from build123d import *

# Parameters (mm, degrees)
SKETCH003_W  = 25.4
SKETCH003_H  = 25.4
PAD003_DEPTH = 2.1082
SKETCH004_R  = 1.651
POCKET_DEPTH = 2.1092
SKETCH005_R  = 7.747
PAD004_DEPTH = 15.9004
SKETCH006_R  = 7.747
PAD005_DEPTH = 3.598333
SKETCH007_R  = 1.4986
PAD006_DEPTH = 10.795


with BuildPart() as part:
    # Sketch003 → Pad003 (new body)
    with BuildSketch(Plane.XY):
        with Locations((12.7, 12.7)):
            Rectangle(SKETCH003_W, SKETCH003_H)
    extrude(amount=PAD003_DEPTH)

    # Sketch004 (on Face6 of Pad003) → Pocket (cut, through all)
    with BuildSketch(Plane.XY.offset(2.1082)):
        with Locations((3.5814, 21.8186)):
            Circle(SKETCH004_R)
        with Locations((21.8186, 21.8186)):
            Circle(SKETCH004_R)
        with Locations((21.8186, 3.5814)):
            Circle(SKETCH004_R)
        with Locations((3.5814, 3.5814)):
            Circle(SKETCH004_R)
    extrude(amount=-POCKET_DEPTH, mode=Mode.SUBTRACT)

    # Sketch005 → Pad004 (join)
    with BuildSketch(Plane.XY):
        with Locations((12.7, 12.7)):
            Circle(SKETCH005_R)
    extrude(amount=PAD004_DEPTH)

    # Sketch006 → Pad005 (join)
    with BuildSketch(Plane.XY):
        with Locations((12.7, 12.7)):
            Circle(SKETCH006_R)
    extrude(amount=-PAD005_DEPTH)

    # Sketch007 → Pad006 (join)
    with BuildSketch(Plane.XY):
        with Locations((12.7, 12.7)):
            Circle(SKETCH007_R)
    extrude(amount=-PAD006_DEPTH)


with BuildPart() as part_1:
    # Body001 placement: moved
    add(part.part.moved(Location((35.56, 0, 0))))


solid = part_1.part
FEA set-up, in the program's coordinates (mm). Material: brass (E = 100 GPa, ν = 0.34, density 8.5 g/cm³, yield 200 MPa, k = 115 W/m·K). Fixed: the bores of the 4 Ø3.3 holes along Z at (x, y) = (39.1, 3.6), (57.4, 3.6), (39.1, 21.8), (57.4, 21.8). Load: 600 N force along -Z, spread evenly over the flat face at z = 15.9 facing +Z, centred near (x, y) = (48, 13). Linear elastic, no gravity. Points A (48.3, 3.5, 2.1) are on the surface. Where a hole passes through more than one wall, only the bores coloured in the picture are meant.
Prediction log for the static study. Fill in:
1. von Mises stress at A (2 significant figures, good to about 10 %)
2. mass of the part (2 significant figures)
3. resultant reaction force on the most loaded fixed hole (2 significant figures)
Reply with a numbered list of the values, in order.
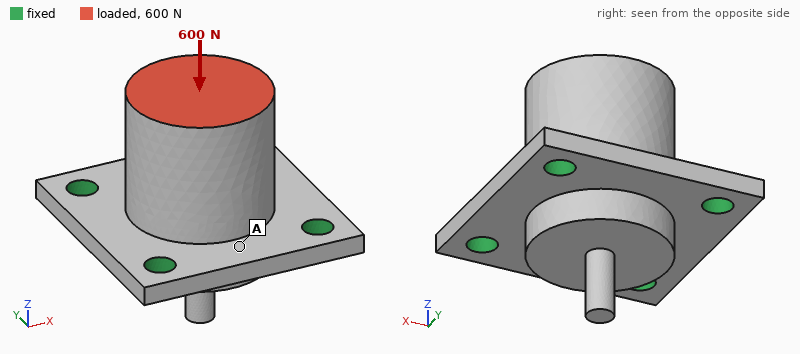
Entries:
1. 12 MPa
2. 39 g
3. 150 N
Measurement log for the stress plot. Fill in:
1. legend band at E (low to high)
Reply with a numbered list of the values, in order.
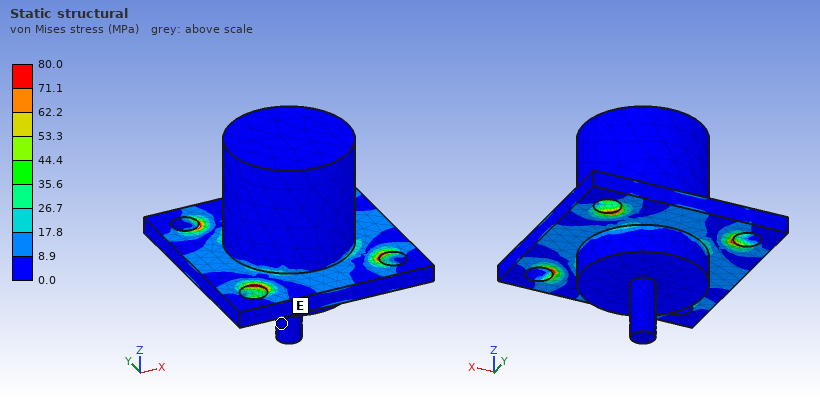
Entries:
1. 0.0 to 8.9 MPa
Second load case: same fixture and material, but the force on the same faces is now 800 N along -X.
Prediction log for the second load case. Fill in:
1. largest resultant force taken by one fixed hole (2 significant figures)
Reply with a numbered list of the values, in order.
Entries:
1. 440 N
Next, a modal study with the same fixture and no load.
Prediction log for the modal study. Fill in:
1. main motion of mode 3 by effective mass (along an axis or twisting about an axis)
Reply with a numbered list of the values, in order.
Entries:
1. along Z
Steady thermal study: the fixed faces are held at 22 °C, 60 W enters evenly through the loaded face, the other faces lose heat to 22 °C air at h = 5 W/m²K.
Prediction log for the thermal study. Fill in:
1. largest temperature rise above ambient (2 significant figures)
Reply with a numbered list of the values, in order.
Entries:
1. 73 K
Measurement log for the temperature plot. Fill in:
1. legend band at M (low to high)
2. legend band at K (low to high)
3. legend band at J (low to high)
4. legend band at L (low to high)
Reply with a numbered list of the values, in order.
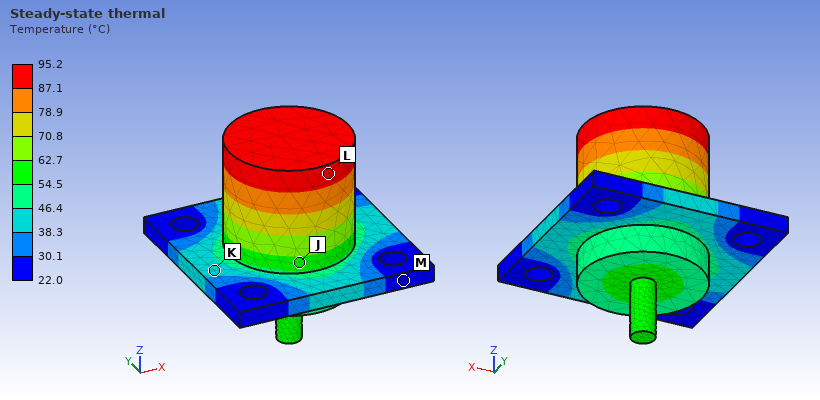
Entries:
1. 22.0 to 30.1 °C
2. 38.3 to 46.4 °C
3. 54.5 to 62.7 °C
4. 87.1 to 95.2 °C
